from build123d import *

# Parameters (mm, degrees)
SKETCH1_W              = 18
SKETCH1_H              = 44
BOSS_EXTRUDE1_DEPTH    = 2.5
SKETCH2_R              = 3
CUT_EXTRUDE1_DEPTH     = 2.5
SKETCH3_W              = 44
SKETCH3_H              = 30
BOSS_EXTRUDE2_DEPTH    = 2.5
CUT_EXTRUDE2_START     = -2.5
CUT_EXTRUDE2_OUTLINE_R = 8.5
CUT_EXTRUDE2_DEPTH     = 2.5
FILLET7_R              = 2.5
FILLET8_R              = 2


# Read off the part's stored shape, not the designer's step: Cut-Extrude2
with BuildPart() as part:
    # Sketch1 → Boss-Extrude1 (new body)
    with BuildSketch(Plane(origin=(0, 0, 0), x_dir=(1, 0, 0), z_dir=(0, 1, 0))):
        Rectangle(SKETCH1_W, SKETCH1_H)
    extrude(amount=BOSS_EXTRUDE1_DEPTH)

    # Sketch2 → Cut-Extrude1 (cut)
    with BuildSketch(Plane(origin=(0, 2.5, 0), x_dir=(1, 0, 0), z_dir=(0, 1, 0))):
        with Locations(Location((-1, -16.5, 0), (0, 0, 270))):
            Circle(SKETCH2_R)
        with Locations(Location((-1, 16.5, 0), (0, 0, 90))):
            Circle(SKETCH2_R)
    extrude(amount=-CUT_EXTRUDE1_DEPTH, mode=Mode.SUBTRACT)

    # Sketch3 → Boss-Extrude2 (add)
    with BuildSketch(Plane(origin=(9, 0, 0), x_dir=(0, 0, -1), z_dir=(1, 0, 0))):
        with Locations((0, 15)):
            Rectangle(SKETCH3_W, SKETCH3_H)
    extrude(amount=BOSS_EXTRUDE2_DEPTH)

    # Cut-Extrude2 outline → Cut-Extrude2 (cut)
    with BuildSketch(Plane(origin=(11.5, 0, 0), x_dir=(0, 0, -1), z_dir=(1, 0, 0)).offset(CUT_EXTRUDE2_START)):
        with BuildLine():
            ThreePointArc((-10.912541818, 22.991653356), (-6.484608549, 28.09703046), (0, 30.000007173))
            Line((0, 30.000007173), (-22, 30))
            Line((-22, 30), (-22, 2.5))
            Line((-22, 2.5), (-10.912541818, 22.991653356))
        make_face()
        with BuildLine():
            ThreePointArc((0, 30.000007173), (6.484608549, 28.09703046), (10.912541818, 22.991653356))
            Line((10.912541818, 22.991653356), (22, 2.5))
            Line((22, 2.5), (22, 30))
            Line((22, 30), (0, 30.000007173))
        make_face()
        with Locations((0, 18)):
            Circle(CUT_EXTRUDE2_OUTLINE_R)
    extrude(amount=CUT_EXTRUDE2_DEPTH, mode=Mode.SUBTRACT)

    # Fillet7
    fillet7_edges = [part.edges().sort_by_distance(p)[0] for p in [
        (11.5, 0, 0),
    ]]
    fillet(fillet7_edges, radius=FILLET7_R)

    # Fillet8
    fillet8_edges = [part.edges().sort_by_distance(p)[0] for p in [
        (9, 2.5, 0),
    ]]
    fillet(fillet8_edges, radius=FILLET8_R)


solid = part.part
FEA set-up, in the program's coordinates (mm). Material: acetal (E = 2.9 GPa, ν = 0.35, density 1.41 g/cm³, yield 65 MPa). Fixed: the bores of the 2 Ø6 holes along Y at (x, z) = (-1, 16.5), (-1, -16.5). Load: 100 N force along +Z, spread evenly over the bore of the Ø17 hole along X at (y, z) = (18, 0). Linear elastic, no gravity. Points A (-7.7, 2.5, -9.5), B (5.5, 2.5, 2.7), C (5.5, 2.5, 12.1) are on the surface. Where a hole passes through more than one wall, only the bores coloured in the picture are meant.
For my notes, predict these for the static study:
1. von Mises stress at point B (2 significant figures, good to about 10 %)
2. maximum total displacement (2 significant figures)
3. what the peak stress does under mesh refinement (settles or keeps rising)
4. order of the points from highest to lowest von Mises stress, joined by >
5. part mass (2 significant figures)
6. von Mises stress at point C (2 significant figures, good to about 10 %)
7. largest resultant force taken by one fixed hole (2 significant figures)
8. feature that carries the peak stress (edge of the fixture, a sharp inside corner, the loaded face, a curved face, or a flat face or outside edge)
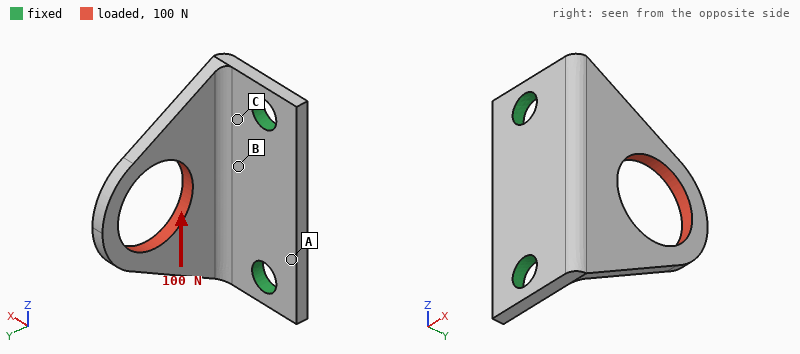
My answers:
5.6 MPa
0.39 mm
keeps rising
C > B > A
4.9 g
9.2 MPa
76 N
edge of the fixture
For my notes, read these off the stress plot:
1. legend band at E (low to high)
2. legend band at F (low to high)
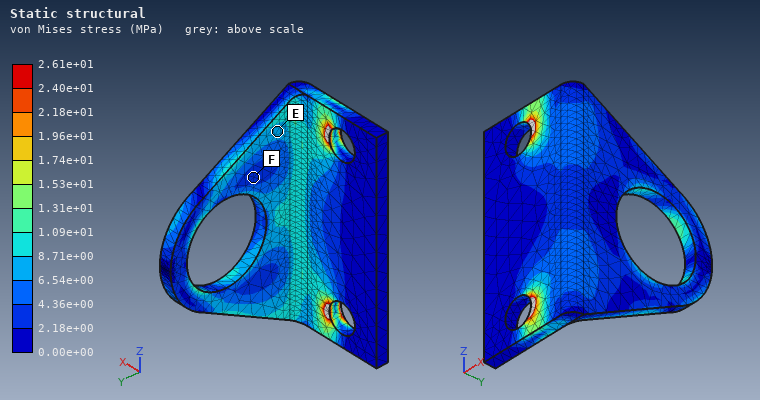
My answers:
6.54e+00 to 8.71e+00 MPa
2.18e+00 to 4.36e+00 MPa
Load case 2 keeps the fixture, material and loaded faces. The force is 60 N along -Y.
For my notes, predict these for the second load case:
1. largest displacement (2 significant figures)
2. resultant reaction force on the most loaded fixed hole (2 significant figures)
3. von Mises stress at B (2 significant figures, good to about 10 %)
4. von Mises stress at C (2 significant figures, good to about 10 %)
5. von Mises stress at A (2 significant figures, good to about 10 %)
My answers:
0.52 mm
30 N
3.3 MPa
6.1 MPa
1.6 MPa
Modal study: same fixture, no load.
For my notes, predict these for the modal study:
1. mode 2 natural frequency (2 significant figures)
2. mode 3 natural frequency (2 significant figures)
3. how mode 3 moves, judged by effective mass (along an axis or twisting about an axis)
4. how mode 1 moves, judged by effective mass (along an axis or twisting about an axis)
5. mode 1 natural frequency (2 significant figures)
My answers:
1900 Hz
2300 Hz
along Y
along X
830 Hz
